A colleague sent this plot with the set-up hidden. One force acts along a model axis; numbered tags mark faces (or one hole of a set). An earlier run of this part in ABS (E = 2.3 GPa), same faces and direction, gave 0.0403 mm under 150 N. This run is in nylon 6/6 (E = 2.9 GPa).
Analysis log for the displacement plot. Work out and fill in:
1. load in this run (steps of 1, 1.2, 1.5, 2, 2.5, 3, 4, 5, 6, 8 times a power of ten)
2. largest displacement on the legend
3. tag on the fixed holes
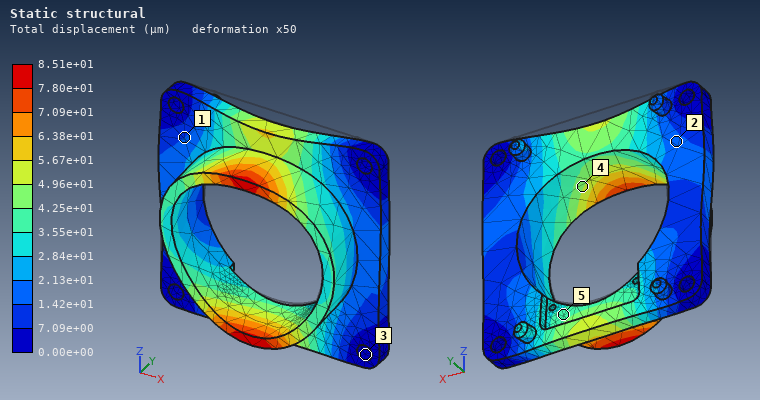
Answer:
400 N
8.51e+01 µm
3
